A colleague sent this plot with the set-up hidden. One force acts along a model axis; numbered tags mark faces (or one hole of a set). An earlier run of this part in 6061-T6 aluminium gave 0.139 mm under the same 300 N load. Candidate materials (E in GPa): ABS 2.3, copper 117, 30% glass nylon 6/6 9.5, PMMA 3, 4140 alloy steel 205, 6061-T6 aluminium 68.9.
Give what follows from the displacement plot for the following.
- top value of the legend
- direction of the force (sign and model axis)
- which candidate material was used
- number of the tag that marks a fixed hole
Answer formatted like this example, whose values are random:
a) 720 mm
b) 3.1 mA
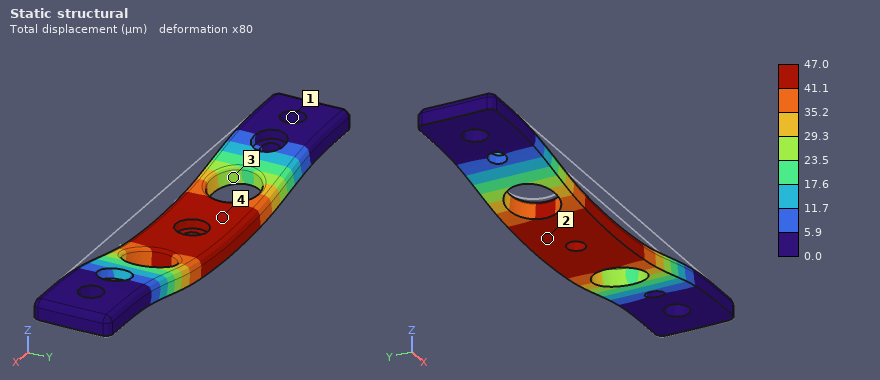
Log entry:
a) 47.0 µm
b) -Z
c) 4140 alloy steel
d) 1
